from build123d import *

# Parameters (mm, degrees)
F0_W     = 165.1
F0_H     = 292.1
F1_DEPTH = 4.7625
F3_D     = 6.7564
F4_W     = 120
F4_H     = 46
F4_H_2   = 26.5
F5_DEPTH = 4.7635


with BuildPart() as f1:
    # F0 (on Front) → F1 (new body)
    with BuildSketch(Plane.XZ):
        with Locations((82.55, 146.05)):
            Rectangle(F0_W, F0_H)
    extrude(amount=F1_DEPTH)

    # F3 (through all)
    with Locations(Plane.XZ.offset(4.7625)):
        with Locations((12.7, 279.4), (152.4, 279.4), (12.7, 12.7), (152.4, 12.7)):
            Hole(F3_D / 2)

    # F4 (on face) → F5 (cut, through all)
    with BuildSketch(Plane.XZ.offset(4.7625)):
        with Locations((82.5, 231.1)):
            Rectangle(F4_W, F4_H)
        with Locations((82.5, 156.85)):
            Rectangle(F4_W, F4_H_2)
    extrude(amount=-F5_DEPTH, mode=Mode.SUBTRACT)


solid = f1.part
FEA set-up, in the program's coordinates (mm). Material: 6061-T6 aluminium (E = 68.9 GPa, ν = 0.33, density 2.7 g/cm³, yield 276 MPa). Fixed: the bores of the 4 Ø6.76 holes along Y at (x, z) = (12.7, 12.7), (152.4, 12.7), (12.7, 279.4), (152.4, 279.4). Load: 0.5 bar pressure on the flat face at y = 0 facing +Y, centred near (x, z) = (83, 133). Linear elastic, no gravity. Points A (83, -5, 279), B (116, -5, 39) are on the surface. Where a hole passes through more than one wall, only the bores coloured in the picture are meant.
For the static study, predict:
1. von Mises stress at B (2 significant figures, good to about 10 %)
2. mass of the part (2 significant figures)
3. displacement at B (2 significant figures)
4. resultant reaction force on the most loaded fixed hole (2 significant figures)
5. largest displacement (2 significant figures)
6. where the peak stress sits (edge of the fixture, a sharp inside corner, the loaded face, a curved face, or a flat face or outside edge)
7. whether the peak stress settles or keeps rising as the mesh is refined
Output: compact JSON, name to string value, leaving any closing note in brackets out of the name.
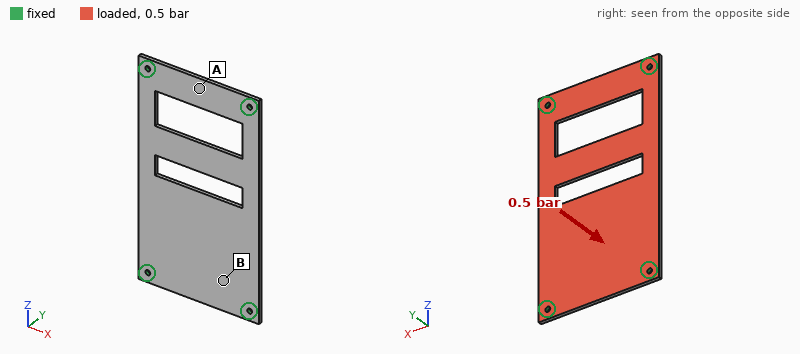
{"von Mises stress at B": "29 MPa", "mass of the part": "510 g", "displacement at B": "0.42 mm", "resultant reaction force on the most loaded fixed hole": "560 N", "largest displacement": "2.3 mm", "where the peak stress sits": "edge of the fixture", "whether the peak stress settles or keeps rising as the mesh is refined": "keeps rising"}
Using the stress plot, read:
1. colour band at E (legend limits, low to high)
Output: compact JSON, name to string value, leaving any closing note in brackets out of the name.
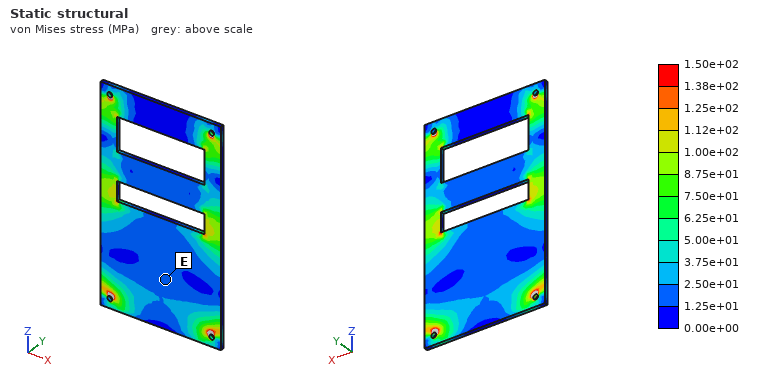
{"colour band at E": "1.25e+01 to 2.50e+01 MPa"}
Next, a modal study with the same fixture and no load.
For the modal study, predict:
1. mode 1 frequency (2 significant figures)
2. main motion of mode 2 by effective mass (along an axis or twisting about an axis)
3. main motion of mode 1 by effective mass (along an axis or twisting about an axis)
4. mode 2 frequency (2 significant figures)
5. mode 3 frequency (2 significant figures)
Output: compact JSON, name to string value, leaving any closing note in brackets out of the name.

{"mode 1 frequency": "250 Hz", "main motion of mode 2 by effective mass": "twisting about Z", "main motion of mode 1 by effective mass": "along Y", "mode 2 frequency": "470 Hz", "mode 3 frequency": "650 Hz"}
